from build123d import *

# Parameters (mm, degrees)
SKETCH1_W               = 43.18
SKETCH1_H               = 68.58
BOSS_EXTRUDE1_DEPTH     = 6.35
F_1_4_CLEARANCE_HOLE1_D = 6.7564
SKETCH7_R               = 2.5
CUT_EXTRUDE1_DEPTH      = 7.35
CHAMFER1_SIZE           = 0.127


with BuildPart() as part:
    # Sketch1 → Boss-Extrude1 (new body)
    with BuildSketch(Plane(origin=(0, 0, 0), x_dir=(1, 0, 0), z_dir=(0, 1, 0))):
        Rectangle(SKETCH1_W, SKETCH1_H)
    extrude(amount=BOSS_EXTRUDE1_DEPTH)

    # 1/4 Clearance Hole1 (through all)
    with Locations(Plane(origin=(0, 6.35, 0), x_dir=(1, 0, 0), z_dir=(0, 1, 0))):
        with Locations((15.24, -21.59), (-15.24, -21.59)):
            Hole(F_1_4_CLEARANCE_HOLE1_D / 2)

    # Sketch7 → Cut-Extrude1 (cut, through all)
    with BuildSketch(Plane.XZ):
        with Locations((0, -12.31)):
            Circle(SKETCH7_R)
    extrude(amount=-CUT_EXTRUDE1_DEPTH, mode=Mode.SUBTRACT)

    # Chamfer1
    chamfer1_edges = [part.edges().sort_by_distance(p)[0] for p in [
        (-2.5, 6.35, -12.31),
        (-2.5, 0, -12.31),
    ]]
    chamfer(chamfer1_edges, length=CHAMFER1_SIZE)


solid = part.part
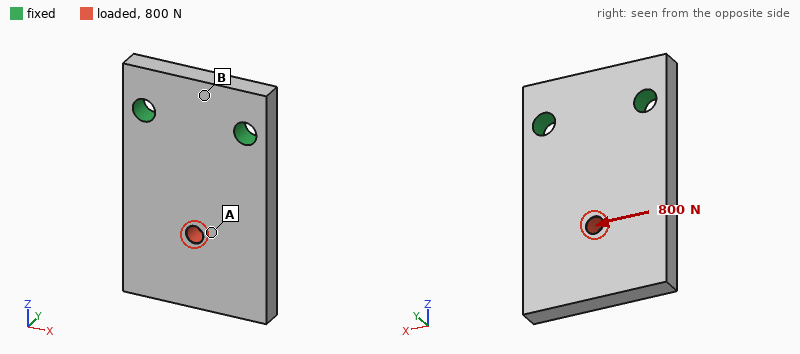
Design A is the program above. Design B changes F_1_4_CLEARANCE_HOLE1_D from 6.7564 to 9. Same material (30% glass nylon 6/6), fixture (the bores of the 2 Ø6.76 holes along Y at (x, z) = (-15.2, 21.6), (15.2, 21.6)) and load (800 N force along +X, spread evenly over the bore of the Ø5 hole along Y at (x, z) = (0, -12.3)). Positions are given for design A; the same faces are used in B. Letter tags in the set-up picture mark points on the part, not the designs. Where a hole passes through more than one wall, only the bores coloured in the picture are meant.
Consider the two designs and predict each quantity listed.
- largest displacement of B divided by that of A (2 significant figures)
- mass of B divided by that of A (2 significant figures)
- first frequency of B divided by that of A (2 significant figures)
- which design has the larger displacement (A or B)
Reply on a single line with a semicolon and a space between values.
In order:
0.91; 0.98; 1.1; A
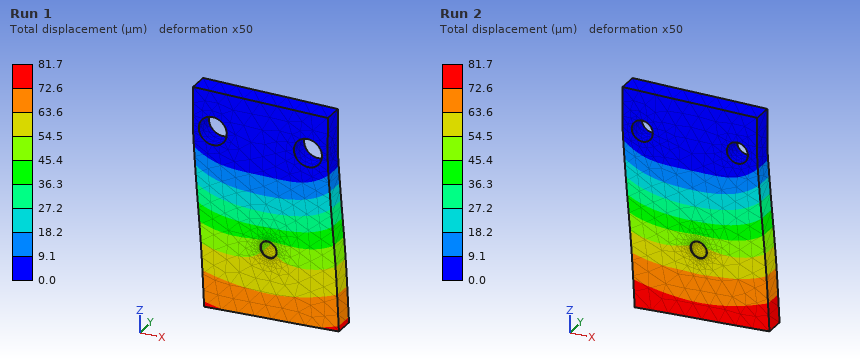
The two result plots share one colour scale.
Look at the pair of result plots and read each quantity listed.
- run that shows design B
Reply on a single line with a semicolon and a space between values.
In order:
Run 1
